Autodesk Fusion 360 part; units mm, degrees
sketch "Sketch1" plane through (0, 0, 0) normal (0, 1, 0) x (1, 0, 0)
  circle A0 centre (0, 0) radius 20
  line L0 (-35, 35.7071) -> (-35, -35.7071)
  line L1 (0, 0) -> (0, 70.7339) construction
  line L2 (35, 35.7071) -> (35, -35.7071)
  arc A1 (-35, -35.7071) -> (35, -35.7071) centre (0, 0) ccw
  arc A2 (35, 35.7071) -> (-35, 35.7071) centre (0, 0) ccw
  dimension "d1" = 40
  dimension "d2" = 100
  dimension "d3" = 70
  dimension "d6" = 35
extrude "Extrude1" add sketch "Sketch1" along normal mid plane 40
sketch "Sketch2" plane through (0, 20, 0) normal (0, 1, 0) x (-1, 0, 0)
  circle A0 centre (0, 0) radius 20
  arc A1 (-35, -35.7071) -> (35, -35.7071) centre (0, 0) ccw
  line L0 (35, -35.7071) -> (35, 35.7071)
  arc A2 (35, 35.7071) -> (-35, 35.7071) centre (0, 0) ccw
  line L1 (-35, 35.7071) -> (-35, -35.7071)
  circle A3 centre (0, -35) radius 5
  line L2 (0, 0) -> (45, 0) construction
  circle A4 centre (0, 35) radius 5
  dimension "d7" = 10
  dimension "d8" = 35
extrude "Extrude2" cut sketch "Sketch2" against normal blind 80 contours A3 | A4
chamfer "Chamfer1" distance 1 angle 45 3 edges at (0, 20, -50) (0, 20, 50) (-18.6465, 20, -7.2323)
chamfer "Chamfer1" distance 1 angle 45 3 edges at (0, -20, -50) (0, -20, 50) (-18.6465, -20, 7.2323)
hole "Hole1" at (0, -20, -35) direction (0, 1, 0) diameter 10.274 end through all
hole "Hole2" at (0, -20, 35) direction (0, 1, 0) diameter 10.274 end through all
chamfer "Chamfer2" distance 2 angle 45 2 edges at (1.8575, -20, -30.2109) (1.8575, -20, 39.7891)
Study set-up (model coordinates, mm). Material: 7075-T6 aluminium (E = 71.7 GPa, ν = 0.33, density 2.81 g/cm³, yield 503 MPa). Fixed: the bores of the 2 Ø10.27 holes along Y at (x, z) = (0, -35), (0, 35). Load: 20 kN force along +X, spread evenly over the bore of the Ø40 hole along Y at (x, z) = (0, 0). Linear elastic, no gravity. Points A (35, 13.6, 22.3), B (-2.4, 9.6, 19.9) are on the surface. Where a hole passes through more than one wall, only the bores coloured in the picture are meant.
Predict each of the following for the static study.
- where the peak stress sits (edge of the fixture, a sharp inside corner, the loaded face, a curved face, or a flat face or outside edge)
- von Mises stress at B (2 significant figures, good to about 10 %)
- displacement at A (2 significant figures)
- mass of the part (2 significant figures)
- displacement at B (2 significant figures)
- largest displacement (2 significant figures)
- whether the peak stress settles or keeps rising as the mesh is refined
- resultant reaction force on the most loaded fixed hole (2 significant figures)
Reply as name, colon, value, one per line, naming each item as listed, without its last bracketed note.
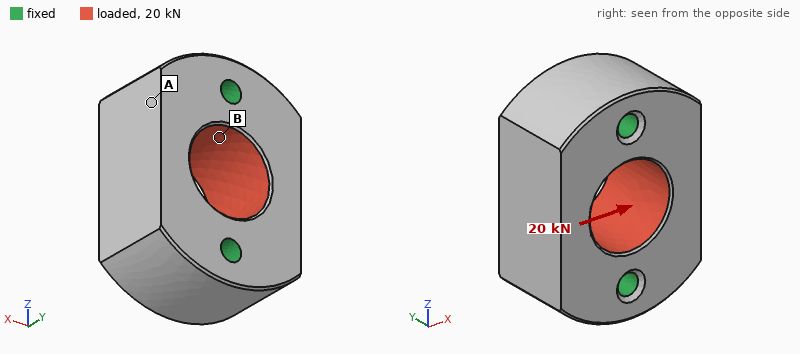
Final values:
where the peak stress sits: edge of the fixture
von Mises stress at B: 7.5 MPa
displacement at A: 3.6 µm
mass of the part: 560 g
displacement at B: 3.0 µm
largest displacement: 6.6 µm
whether the peak stress settles or keeps rising as the mesh is refined: keeps rising
resultant reaction force on the most loaded fixed hole: 10 kN
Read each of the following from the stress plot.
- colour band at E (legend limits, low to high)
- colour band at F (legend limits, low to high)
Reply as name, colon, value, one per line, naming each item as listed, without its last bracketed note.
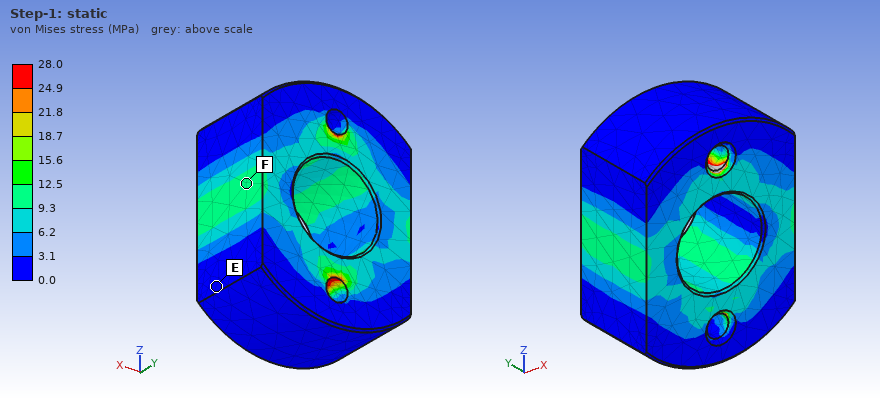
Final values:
colour band at E: 0.0 to 3.1 MPa
colour band at F: 9.3 to 12.5 MPa
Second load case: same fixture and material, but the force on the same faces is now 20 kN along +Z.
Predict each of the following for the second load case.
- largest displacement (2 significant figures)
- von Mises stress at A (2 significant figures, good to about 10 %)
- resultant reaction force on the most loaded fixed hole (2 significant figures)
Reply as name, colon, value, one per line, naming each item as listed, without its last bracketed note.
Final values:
largest displacement: 4.9 µm
von Mises stress at A: 2.4 MPa
resultant reaction force on the most loaded fixed hole: 10 kN
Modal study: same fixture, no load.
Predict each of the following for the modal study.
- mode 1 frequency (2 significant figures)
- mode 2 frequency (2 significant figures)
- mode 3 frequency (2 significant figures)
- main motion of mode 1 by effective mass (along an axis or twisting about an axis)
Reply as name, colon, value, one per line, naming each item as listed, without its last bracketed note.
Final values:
mode 1 frequency: 12 kHz
mode 2 frequency: 13 kHz
mode 3 frequency: 13 kHz
main motion of mode 1 by effective mass: twisting about Z
